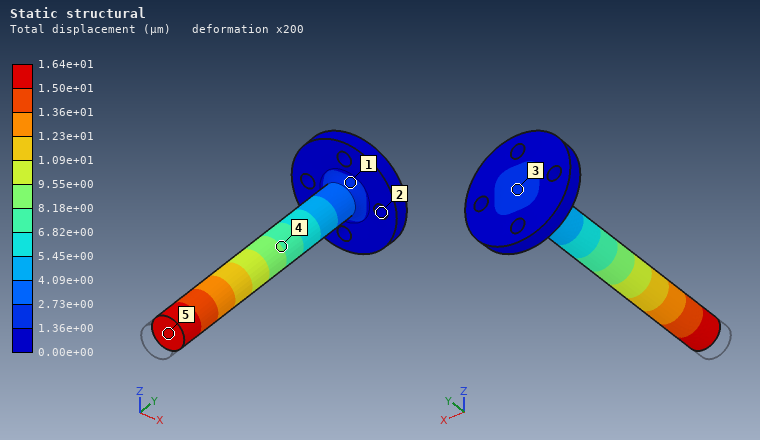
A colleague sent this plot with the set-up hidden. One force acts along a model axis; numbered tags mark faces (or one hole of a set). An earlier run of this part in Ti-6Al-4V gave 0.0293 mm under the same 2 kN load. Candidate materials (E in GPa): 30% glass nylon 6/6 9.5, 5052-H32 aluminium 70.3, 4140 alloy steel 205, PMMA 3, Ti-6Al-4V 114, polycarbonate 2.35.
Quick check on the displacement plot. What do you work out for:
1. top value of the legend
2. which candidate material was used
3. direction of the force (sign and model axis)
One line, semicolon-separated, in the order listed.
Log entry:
1.64e+01 µm; 4140 alloy steel; +Y
